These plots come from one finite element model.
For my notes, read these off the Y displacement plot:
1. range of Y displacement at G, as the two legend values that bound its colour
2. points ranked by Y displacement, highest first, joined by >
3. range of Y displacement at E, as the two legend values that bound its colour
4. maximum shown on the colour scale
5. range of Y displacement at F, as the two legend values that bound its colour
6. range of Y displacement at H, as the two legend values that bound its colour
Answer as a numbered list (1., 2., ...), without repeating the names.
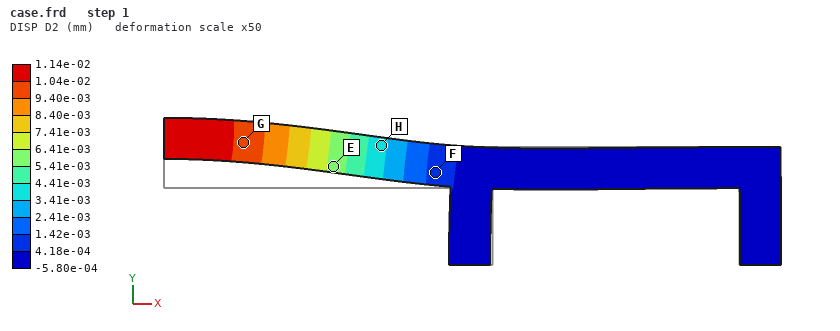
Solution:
1. 9.40e-03 to 1.04e-02 mm
2. G > E > H > F
3. 5.41e-03 to 6.41e-03 mm
4. 1.14e-02 mm
5. 4.18e-04 to 1.42e-03 mm
6. 3.41e-03 to 4.41e-03 mm
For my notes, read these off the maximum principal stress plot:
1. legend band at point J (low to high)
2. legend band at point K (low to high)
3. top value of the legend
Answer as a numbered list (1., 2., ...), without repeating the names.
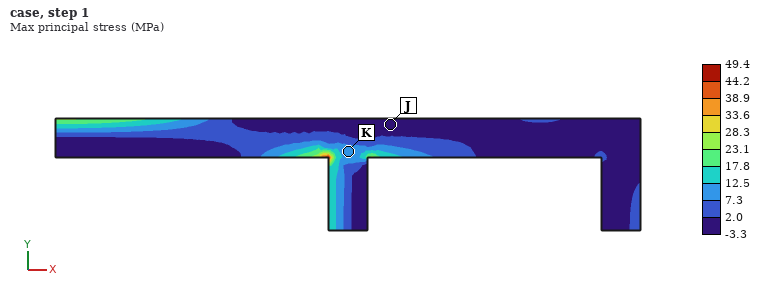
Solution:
1. -3.3 to 2.0 MPa
2. 7.3 to 12.5 MPa
3. 49.4 MPa
